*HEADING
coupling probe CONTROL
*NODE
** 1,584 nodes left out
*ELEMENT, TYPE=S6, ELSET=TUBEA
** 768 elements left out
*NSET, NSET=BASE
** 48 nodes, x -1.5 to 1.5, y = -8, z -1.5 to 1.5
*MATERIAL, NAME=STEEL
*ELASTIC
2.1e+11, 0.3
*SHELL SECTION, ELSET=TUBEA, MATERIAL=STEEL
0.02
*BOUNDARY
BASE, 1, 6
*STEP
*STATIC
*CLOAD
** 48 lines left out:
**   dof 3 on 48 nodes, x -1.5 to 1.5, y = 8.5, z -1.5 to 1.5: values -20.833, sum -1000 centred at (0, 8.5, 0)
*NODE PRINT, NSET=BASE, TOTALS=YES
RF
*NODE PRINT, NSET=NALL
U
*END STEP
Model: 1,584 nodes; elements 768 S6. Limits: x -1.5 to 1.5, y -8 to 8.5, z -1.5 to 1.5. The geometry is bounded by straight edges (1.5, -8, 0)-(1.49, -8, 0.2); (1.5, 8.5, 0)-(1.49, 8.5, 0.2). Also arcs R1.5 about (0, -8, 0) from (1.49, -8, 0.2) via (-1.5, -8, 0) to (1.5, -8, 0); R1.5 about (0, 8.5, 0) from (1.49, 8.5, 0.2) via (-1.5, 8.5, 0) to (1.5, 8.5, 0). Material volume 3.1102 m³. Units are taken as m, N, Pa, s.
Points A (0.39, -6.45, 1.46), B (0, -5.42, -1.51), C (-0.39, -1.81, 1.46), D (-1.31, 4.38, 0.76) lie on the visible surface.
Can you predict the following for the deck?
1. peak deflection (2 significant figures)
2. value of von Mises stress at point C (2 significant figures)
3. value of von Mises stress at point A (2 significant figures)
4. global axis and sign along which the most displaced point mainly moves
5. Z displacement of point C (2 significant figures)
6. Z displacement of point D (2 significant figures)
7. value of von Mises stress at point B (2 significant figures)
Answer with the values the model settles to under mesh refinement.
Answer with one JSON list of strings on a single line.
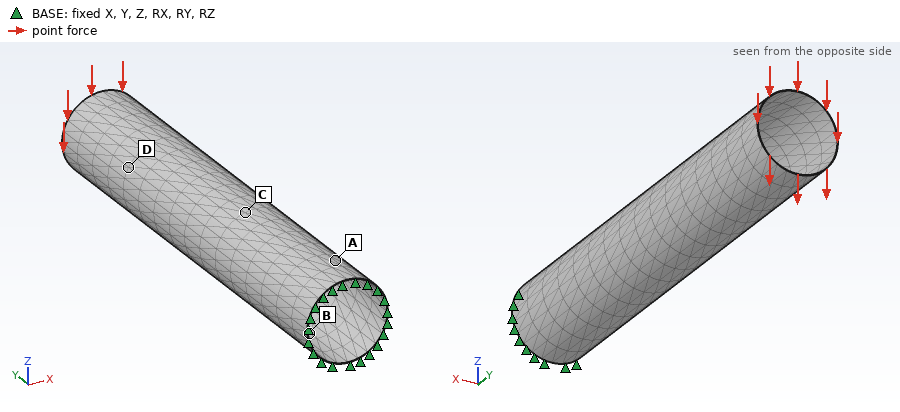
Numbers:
["3.7e-05 m", "71000 Pa", "1.0e+05 Pa", "-Z", "-7.1e-06 m", "-2.3e-05 m", "99000 Pa"]
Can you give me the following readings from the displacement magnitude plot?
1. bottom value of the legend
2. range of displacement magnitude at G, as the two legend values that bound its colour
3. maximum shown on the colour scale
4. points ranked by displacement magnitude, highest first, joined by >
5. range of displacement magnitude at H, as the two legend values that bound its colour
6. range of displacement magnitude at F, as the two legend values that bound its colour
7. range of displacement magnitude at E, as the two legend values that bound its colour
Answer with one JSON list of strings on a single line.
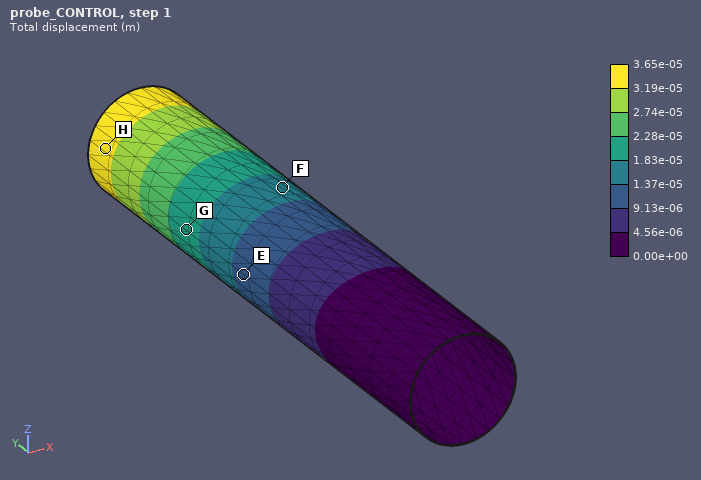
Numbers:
["0.00e+00 m", "1.83e-05 to 2.28e-05 m", "3.65e-05 m", "H > G > F > E", "3.19e-05 to 3.65e-05 m", "1.37e-05 to 1.83e-05 m", "9.13e-06 to 1.37e-05 m"]
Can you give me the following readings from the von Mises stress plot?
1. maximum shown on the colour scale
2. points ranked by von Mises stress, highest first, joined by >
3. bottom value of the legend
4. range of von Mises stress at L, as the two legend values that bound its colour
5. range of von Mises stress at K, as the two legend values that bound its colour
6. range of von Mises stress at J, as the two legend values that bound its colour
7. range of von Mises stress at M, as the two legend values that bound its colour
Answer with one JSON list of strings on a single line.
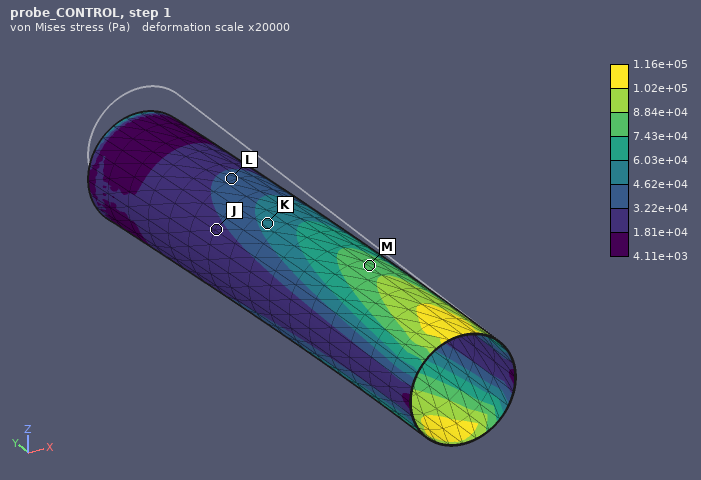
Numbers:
["1.16e+05 Pa", "M > K > L > J", "4.11e+03 Pa", "3.22e+04 to 4.62e+04 Pa", "4.62e+04 to 6.03e+04 Pa", "1.81e+04 to 3.22e+04 Pa", "7.43e+04 to 8.84e+04 Pa"]
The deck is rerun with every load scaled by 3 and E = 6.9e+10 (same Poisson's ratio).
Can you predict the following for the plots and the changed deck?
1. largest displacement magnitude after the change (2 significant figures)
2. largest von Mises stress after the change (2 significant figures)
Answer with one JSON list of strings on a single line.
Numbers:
["3.3e-04 m", "3.5e+05 Pa"]
